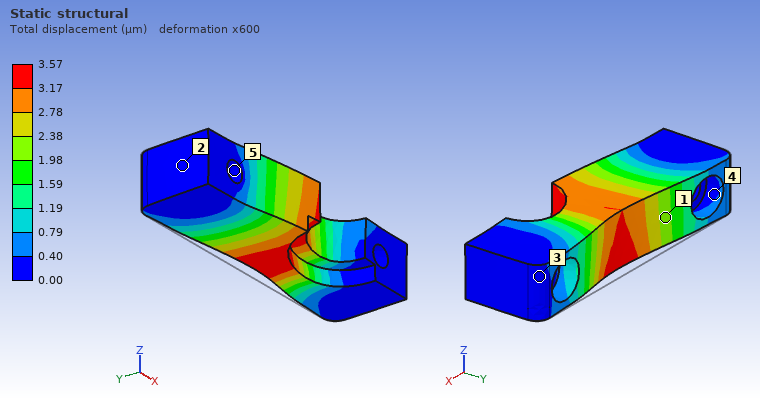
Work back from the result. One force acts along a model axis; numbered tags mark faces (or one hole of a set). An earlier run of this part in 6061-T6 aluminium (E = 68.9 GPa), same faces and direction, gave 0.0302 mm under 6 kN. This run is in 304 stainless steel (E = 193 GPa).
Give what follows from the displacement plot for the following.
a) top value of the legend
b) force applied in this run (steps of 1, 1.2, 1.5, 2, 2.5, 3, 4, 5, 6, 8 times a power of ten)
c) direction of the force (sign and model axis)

3.57 µm
2 kN
-Y
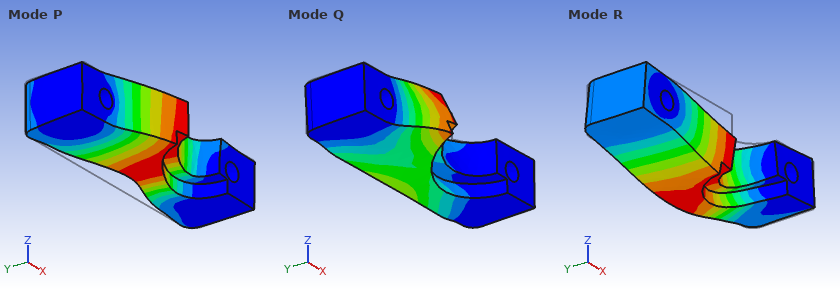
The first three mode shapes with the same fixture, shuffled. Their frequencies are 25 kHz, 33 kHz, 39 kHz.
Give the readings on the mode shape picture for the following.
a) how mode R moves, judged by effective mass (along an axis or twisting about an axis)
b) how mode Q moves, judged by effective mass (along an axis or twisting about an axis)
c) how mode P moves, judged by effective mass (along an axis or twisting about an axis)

along Z
twisting about X
along Y
